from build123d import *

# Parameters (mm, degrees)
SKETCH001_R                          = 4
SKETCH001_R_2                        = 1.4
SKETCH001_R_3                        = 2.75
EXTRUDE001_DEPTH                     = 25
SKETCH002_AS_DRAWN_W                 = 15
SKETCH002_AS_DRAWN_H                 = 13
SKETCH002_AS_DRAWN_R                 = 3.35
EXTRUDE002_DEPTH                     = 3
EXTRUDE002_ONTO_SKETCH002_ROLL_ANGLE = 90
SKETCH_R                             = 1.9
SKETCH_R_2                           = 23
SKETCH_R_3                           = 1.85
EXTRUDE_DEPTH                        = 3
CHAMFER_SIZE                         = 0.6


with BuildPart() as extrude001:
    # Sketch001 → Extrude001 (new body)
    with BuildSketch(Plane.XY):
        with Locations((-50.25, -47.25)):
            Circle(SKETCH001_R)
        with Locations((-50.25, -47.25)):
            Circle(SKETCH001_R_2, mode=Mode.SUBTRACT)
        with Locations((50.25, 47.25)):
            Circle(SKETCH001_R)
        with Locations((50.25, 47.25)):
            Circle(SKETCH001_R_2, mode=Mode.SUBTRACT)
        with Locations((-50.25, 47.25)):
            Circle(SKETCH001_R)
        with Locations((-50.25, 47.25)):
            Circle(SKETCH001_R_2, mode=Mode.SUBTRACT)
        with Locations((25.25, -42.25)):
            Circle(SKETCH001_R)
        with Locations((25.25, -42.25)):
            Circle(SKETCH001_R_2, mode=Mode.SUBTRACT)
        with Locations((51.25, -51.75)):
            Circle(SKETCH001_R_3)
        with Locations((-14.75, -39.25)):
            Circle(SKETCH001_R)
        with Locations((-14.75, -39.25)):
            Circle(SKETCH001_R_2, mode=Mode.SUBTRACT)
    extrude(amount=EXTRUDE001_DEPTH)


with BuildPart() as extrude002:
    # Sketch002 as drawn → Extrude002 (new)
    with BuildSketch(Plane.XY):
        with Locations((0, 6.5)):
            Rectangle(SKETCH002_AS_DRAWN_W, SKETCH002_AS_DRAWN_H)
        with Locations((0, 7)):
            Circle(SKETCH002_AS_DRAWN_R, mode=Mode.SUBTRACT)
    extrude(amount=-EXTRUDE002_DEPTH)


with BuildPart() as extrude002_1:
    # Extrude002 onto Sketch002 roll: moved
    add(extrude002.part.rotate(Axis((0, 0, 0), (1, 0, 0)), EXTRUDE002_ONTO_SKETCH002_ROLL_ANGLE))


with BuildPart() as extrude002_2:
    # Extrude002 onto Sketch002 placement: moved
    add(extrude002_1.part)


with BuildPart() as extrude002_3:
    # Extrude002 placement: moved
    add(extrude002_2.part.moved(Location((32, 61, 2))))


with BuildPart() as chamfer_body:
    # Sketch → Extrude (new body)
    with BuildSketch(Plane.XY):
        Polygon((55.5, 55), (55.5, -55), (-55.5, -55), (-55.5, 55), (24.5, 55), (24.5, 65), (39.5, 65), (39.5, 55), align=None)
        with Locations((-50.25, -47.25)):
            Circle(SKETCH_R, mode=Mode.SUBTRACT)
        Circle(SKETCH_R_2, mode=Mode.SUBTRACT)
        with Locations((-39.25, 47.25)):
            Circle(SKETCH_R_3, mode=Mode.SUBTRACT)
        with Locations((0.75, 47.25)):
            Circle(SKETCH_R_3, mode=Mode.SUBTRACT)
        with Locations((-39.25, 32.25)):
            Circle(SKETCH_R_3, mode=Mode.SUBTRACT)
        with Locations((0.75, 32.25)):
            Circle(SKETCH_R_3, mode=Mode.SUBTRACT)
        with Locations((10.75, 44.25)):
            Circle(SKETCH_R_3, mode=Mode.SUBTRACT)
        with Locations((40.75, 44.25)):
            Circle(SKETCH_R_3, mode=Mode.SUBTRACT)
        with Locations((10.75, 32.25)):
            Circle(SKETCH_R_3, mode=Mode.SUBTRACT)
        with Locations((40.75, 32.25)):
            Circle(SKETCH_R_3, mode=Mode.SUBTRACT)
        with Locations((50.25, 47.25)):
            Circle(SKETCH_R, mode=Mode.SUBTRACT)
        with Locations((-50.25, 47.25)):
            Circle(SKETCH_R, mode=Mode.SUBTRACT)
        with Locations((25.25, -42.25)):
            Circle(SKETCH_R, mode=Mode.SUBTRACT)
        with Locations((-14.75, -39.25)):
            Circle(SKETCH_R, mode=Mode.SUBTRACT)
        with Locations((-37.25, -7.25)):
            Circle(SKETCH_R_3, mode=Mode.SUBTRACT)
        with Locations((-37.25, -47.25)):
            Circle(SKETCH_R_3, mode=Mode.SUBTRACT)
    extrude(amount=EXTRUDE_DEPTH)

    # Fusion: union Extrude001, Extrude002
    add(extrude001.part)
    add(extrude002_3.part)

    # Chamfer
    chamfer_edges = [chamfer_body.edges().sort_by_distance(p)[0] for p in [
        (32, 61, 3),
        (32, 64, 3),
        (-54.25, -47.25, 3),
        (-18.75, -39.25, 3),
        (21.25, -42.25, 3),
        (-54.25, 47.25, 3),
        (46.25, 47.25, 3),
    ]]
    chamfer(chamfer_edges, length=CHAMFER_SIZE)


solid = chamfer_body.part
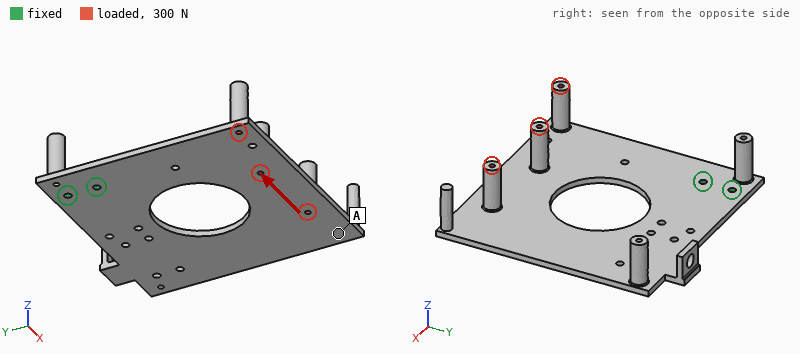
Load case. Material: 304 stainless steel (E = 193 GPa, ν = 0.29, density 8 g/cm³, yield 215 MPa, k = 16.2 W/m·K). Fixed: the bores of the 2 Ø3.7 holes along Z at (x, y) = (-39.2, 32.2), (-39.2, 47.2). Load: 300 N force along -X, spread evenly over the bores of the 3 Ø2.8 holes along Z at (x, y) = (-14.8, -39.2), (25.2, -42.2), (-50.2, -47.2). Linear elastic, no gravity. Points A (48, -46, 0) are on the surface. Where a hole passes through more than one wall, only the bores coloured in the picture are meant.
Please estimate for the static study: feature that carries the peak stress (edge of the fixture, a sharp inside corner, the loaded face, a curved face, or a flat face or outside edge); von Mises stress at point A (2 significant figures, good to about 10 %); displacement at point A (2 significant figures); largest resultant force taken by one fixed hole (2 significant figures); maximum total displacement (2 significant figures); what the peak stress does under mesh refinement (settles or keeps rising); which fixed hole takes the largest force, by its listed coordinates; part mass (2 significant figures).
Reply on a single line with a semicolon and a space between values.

edge of the fixture; 6.4 MPa; 0.54 mm; 1.6 kN; 0.62 mm; keeps rising; (-39.2, 32.2); 300 g
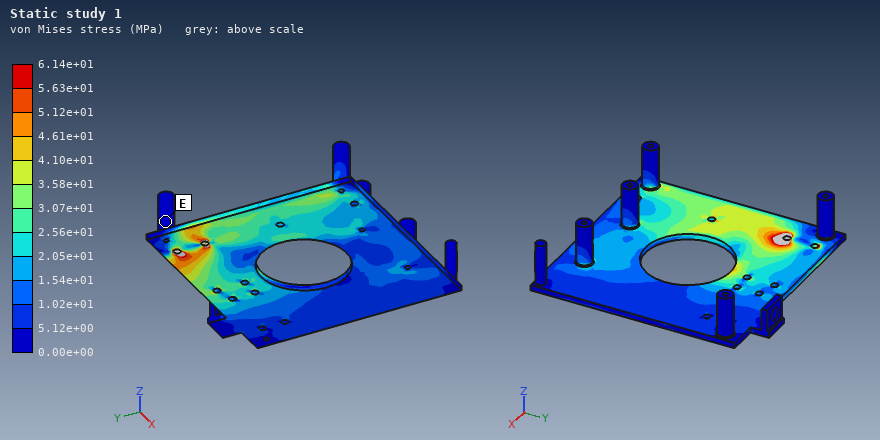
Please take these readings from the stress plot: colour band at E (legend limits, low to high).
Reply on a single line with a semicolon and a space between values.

0.00e+00 to 5.12e+00 MPa
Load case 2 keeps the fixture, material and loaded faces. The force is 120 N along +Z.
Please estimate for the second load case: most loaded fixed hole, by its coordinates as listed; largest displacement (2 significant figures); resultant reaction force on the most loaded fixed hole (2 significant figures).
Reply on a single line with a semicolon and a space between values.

(-39.2, 32.2); 1.4 mm; 430 N
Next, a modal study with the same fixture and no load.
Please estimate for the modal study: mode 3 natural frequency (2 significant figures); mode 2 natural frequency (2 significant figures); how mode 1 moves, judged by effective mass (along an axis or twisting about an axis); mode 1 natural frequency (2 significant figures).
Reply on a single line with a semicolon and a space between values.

490 Hz; 230 Hz; along Z; 130 Hz
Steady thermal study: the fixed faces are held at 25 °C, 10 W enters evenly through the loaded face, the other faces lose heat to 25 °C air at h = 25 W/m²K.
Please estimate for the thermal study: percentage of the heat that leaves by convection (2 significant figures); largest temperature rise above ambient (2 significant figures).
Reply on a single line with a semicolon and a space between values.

97 %; 79 K
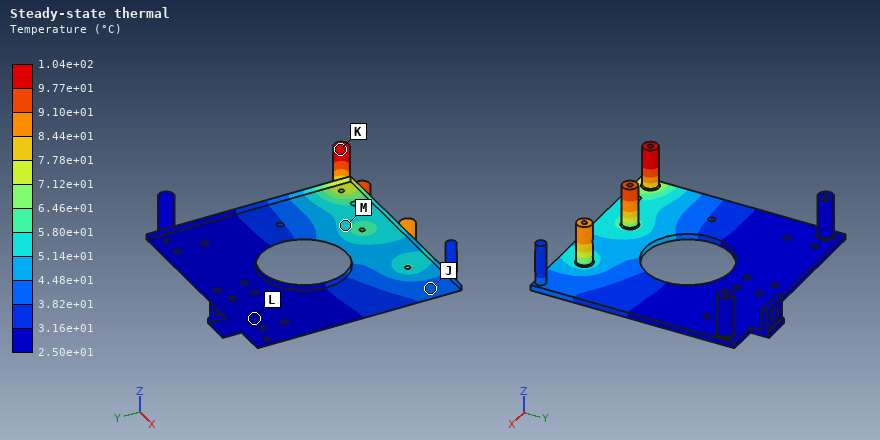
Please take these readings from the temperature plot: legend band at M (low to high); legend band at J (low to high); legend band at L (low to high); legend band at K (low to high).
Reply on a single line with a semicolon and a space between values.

5.14e+01 to 5.80e+01 °C; 3.82e+01 to 4.48e+01 °C; 2.50e+01 to 3.16e+01 °C; 9.77e+01 to 1.04e+02 °C
